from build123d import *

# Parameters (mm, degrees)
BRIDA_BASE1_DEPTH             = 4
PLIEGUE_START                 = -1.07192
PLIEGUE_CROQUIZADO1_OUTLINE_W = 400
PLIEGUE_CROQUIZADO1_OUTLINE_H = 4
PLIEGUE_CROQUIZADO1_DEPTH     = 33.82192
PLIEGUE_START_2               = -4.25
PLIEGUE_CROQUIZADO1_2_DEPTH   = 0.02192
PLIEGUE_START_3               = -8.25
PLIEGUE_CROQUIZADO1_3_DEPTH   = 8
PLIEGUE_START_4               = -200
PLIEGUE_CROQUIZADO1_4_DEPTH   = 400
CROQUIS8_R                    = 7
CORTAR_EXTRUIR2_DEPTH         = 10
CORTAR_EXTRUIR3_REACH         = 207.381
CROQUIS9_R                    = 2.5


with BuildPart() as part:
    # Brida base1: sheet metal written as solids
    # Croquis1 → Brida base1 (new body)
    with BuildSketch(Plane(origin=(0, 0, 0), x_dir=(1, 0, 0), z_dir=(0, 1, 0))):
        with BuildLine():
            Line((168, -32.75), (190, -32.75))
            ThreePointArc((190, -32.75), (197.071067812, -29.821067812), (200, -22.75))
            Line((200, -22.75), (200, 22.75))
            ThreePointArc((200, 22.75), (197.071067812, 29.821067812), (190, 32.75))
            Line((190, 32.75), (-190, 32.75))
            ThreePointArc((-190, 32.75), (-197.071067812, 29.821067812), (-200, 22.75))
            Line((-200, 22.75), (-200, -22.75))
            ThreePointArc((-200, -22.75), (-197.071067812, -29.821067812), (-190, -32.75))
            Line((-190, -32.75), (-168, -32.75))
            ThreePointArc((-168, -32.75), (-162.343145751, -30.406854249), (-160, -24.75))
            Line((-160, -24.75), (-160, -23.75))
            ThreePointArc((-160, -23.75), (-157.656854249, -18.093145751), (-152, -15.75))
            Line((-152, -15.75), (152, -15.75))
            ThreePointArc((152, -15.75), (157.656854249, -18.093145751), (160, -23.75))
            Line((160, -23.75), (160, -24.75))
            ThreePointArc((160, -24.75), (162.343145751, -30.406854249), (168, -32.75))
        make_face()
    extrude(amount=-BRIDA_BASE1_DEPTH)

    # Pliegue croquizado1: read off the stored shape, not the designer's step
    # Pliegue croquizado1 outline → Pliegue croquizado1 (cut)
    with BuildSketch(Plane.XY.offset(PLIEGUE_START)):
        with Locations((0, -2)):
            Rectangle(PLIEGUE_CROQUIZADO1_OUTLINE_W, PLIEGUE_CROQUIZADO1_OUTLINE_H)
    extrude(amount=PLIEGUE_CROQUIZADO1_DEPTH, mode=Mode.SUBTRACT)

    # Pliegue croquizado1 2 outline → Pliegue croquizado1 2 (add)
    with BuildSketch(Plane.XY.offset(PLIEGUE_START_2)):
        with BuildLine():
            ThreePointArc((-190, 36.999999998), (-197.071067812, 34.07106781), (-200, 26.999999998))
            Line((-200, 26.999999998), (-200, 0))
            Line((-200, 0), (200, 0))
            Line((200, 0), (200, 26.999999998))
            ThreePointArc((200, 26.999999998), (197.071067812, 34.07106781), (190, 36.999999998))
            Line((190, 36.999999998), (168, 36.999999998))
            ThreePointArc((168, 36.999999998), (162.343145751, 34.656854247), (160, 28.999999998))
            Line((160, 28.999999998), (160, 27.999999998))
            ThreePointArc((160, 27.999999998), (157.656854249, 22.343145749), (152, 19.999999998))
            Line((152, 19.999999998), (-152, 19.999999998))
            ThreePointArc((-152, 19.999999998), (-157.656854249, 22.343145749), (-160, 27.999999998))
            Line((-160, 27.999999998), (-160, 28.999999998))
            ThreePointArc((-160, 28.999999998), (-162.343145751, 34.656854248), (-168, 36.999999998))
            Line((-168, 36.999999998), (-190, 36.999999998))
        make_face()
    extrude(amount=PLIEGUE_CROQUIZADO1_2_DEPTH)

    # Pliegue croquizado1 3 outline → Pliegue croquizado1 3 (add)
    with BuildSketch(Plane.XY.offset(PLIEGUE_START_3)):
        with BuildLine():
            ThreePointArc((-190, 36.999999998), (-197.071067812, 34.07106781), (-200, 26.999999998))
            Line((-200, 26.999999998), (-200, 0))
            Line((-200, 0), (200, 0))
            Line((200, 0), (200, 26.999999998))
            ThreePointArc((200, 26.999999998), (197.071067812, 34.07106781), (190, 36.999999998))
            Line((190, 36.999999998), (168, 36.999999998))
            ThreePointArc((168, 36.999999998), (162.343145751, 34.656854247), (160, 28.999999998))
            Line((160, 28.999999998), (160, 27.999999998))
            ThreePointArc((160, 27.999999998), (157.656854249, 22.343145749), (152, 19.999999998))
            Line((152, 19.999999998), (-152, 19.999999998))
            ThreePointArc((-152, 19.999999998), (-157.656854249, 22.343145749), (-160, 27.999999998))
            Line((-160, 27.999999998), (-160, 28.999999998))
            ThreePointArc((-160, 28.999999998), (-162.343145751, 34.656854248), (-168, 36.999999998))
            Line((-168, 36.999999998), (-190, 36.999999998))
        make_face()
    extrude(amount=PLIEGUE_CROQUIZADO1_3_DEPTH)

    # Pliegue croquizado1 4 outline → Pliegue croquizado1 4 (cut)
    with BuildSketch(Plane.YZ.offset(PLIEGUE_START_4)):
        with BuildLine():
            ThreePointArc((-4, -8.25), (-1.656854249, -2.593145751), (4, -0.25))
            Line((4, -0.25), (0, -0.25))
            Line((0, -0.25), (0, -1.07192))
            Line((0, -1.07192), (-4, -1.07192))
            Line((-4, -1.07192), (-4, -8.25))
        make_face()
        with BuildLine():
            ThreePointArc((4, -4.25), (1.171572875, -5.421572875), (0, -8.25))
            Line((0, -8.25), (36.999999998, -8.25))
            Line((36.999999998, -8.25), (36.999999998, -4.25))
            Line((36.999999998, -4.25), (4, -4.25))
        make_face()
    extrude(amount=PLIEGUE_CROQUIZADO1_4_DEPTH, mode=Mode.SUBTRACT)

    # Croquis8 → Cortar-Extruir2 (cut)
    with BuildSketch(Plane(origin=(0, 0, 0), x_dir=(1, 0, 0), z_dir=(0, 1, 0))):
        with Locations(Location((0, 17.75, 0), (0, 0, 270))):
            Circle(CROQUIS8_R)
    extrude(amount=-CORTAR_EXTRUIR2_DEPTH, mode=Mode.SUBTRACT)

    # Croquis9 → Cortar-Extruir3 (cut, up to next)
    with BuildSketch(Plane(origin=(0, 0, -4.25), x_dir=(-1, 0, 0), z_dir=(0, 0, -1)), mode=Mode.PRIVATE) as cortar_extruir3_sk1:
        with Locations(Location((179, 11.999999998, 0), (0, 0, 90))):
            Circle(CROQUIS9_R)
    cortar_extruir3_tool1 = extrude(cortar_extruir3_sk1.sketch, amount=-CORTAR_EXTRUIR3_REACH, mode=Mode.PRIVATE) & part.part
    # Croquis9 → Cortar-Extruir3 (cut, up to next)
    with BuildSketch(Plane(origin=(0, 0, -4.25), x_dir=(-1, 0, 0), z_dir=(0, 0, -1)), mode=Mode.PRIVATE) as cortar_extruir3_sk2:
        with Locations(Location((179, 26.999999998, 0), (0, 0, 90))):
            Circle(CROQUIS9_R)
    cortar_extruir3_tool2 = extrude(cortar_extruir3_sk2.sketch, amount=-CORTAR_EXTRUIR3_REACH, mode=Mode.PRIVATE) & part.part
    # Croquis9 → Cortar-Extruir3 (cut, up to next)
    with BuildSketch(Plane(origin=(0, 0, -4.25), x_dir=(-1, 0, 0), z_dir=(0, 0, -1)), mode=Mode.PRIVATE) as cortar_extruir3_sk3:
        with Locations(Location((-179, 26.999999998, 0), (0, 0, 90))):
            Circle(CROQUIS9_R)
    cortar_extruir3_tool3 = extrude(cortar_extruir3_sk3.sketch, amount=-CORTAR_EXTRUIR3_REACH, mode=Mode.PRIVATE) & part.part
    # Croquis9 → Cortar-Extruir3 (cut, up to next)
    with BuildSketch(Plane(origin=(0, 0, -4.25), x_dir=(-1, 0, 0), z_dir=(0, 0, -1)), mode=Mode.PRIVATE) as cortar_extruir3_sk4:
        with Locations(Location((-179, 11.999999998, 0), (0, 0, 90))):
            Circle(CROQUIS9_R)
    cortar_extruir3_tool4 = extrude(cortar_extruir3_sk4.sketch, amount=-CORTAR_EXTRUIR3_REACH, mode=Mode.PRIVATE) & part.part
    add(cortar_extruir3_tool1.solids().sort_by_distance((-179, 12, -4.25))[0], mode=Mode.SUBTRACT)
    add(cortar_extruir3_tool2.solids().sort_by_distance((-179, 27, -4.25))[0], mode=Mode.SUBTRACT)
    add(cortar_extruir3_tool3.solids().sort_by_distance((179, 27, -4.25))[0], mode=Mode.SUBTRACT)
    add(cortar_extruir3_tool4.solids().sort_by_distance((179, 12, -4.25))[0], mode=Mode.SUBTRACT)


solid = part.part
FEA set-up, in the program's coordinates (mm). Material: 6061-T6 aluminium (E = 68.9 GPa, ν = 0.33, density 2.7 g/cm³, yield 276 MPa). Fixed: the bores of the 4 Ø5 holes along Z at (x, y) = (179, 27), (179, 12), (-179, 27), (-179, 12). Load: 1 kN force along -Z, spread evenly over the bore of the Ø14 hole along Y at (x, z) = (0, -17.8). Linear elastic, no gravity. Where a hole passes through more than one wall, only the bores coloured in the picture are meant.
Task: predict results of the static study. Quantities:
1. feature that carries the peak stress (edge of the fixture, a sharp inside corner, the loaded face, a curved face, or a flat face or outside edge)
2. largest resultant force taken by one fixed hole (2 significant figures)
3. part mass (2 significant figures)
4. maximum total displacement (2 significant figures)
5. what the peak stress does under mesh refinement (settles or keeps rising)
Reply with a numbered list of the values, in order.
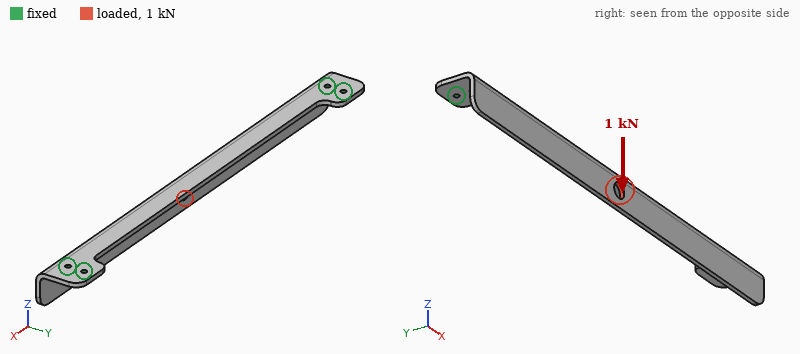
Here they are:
1. edge of the fixture
2. 2.8 kN
3. 230 g
4. 0.80 mm
5. keeps rising
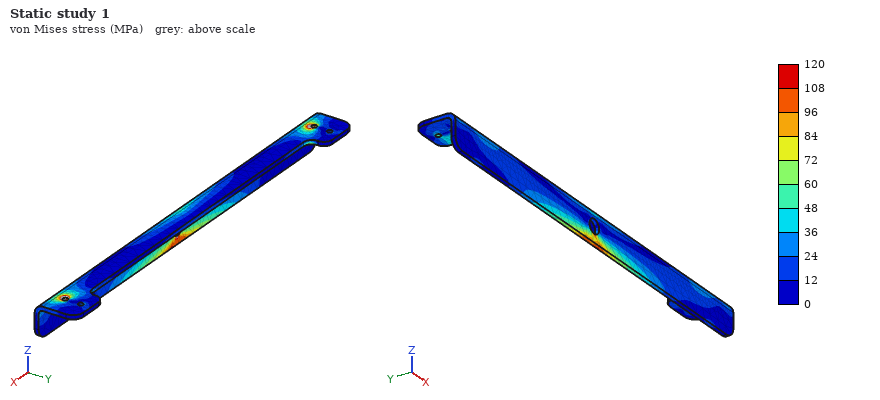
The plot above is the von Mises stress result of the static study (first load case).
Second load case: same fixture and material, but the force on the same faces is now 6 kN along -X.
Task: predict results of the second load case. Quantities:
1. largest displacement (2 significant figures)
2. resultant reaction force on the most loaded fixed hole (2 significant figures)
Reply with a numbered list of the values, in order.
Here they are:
1. 59 µm
2. 3.1 kN
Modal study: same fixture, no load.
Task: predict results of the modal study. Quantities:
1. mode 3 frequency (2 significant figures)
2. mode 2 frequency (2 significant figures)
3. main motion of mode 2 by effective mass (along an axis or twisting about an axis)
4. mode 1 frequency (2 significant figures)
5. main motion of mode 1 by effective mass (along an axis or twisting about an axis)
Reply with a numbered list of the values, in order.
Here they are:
1. 1200 Hz
2. 660 Hz
3. along Z
4. 550 Hz
5. along Y
